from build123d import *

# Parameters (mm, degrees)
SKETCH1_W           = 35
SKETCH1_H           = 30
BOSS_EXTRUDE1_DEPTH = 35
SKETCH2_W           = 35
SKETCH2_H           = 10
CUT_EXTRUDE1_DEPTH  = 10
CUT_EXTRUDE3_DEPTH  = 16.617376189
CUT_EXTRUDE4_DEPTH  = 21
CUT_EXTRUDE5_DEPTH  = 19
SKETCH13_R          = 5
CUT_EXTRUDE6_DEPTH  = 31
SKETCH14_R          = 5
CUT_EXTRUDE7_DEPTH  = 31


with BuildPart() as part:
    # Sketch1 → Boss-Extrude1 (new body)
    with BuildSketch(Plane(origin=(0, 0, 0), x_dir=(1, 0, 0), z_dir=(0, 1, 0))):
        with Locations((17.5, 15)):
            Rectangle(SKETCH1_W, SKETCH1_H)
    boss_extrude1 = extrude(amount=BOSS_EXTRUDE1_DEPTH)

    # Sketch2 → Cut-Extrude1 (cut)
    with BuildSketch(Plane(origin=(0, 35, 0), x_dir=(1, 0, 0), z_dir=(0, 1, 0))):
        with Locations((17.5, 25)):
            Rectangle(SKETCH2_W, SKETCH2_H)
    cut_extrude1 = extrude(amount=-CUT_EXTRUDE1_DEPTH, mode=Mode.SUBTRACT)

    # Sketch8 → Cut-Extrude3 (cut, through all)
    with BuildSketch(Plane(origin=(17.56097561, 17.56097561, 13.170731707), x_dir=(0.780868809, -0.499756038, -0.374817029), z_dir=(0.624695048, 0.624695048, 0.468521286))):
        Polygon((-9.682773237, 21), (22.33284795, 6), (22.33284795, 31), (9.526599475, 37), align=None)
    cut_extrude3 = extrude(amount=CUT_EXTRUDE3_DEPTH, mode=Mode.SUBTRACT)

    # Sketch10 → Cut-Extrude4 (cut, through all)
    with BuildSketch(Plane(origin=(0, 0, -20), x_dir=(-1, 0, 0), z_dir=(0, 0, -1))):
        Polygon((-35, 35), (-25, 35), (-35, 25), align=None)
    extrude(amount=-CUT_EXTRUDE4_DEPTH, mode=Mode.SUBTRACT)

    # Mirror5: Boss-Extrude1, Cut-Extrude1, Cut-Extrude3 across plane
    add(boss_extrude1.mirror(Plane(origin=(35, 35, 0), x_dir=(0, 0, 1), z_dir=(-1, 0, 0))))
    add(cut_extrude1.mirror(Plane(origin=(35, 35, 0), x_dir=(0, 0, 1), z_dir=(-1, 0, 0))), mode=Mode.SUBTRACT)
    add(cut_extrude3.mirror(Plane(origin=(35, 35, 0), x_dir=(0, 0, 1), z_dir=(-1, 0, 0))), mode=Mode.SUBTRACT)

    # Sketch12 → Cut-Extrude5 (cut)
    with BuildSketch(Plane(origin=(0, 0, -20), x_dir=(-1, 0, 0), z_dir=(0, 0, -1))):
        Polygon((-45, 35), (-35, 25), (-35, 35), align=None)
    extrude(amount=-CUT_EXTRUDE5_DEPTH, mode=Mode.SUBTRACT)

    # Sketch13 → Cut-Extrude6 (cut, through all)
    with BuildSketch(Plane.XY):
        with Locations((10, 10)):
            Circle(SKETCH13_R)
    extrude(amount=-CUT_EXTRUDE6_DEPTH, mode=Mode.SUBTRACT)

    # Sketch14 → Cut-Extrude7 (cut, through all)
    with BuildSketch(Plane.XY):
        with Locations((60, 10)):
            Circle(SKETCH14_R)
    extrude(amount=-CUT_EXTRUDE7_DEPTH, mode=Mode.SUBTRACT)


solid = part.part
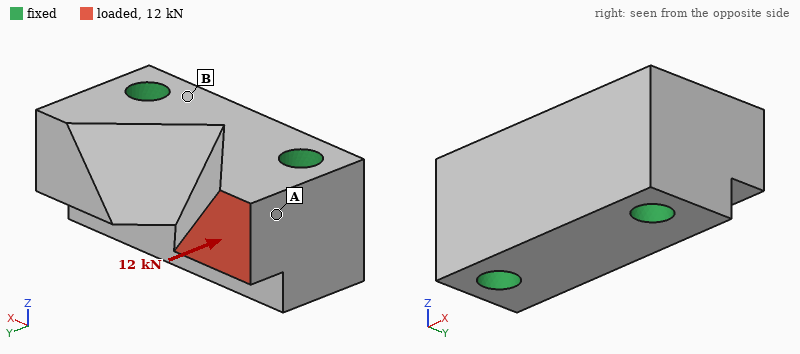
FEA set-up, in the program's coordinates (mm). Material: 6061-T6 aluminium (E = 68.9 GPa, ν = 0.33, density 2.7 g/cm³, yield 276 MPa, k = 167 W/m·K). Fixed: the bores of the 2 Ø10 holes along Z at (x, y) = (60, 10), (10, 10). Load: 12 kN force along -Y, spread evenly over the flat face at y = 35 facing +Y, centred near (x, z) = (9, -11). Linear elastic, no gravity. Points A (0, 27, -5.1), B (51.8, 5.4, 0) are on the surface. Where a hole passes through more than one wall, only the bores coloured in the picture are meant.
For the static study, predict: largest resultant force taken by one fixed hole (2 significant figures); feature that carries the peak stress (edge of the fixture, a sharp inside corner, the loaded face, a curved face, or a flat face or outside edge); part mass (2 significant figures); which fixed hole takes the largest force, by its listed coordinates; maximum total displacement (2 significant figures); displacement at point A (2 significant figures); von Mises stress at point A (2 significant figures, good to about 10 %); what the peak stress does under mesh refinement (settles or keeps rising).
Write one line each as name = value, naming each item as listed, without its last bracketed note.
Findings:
largest resultant force taken by one fixed hole = 12 kN
feature that carries the peak stress = edge of the fixture
part mass = 150 g
which fixed hole takes the largest force, by its listed coordinates = (10, 10)
maximum total displacement = 15 µm
displacement at point A = 9.9 µm
von Mises stress at point A = 36 MPa
what the peak stress does under mesh refinement = keeps rising
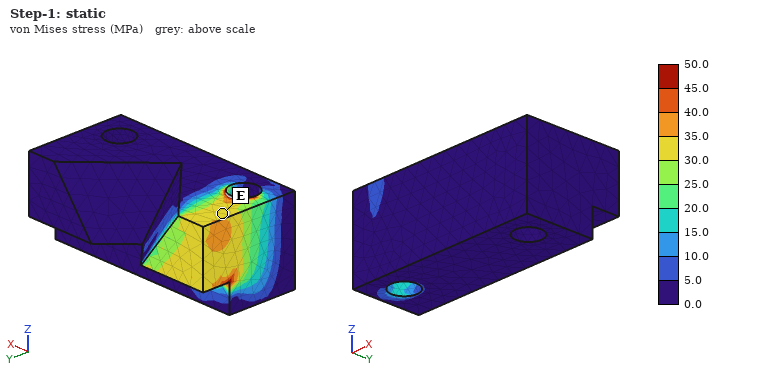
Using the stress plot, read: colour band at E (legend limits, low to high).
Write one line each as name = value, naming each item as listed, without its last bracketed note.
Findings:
colour band at E = 30.0 to 35.0 MPa
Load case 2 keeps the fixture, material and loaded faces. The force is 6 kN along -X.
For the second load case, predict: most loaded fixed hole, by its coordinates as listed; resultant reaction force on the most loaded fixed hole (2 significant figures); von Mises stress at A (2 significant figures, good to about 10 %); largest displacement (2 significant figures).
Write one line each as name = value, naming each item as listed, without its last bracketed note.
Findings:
most loaded fixed hole, by its coordinates as listed = (10, 10)
resultant reaction force on the most loaded fixed hole = 4.6 kN
von Mises stress at A = 29 MPa
largest displacement = 27 µm
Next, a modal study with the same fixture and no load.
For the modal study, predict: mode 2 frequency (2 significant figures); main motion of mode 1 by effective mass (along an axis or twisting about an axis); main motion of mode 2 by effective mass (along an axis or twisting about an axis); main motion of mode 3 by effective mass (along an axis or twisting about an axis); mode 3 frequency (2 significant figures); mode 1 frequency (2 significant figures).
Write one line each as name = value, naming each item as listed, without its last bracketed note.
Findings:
mode 2 frequency = 26 kHz
main motion of mode 1 by effective mass = along Y
main motion of mode 2 by effective mass = along Z
main motion of mode 3 by effective mass = along X
mode 3 frequency = 30 kHz
mode 1 frequency = 22 kHz
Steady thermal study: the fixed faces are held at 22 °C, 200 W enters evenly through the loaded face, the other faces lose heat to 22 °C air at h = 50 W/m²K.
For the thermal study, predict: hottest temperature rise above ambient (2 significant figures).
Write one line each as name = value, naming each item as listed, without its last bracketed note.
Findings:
hottest temperature rise above ambient = 57 K
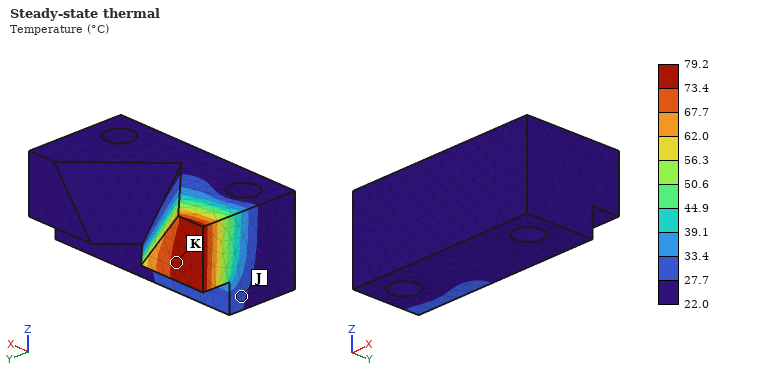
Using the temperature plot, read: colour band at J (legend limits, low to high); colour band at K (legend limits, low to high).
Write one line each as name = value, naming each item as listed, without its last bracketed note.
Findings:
colour band at J = 27.7 to 33.4 °C
colour band at K = 73.4 to 79.2 °C
